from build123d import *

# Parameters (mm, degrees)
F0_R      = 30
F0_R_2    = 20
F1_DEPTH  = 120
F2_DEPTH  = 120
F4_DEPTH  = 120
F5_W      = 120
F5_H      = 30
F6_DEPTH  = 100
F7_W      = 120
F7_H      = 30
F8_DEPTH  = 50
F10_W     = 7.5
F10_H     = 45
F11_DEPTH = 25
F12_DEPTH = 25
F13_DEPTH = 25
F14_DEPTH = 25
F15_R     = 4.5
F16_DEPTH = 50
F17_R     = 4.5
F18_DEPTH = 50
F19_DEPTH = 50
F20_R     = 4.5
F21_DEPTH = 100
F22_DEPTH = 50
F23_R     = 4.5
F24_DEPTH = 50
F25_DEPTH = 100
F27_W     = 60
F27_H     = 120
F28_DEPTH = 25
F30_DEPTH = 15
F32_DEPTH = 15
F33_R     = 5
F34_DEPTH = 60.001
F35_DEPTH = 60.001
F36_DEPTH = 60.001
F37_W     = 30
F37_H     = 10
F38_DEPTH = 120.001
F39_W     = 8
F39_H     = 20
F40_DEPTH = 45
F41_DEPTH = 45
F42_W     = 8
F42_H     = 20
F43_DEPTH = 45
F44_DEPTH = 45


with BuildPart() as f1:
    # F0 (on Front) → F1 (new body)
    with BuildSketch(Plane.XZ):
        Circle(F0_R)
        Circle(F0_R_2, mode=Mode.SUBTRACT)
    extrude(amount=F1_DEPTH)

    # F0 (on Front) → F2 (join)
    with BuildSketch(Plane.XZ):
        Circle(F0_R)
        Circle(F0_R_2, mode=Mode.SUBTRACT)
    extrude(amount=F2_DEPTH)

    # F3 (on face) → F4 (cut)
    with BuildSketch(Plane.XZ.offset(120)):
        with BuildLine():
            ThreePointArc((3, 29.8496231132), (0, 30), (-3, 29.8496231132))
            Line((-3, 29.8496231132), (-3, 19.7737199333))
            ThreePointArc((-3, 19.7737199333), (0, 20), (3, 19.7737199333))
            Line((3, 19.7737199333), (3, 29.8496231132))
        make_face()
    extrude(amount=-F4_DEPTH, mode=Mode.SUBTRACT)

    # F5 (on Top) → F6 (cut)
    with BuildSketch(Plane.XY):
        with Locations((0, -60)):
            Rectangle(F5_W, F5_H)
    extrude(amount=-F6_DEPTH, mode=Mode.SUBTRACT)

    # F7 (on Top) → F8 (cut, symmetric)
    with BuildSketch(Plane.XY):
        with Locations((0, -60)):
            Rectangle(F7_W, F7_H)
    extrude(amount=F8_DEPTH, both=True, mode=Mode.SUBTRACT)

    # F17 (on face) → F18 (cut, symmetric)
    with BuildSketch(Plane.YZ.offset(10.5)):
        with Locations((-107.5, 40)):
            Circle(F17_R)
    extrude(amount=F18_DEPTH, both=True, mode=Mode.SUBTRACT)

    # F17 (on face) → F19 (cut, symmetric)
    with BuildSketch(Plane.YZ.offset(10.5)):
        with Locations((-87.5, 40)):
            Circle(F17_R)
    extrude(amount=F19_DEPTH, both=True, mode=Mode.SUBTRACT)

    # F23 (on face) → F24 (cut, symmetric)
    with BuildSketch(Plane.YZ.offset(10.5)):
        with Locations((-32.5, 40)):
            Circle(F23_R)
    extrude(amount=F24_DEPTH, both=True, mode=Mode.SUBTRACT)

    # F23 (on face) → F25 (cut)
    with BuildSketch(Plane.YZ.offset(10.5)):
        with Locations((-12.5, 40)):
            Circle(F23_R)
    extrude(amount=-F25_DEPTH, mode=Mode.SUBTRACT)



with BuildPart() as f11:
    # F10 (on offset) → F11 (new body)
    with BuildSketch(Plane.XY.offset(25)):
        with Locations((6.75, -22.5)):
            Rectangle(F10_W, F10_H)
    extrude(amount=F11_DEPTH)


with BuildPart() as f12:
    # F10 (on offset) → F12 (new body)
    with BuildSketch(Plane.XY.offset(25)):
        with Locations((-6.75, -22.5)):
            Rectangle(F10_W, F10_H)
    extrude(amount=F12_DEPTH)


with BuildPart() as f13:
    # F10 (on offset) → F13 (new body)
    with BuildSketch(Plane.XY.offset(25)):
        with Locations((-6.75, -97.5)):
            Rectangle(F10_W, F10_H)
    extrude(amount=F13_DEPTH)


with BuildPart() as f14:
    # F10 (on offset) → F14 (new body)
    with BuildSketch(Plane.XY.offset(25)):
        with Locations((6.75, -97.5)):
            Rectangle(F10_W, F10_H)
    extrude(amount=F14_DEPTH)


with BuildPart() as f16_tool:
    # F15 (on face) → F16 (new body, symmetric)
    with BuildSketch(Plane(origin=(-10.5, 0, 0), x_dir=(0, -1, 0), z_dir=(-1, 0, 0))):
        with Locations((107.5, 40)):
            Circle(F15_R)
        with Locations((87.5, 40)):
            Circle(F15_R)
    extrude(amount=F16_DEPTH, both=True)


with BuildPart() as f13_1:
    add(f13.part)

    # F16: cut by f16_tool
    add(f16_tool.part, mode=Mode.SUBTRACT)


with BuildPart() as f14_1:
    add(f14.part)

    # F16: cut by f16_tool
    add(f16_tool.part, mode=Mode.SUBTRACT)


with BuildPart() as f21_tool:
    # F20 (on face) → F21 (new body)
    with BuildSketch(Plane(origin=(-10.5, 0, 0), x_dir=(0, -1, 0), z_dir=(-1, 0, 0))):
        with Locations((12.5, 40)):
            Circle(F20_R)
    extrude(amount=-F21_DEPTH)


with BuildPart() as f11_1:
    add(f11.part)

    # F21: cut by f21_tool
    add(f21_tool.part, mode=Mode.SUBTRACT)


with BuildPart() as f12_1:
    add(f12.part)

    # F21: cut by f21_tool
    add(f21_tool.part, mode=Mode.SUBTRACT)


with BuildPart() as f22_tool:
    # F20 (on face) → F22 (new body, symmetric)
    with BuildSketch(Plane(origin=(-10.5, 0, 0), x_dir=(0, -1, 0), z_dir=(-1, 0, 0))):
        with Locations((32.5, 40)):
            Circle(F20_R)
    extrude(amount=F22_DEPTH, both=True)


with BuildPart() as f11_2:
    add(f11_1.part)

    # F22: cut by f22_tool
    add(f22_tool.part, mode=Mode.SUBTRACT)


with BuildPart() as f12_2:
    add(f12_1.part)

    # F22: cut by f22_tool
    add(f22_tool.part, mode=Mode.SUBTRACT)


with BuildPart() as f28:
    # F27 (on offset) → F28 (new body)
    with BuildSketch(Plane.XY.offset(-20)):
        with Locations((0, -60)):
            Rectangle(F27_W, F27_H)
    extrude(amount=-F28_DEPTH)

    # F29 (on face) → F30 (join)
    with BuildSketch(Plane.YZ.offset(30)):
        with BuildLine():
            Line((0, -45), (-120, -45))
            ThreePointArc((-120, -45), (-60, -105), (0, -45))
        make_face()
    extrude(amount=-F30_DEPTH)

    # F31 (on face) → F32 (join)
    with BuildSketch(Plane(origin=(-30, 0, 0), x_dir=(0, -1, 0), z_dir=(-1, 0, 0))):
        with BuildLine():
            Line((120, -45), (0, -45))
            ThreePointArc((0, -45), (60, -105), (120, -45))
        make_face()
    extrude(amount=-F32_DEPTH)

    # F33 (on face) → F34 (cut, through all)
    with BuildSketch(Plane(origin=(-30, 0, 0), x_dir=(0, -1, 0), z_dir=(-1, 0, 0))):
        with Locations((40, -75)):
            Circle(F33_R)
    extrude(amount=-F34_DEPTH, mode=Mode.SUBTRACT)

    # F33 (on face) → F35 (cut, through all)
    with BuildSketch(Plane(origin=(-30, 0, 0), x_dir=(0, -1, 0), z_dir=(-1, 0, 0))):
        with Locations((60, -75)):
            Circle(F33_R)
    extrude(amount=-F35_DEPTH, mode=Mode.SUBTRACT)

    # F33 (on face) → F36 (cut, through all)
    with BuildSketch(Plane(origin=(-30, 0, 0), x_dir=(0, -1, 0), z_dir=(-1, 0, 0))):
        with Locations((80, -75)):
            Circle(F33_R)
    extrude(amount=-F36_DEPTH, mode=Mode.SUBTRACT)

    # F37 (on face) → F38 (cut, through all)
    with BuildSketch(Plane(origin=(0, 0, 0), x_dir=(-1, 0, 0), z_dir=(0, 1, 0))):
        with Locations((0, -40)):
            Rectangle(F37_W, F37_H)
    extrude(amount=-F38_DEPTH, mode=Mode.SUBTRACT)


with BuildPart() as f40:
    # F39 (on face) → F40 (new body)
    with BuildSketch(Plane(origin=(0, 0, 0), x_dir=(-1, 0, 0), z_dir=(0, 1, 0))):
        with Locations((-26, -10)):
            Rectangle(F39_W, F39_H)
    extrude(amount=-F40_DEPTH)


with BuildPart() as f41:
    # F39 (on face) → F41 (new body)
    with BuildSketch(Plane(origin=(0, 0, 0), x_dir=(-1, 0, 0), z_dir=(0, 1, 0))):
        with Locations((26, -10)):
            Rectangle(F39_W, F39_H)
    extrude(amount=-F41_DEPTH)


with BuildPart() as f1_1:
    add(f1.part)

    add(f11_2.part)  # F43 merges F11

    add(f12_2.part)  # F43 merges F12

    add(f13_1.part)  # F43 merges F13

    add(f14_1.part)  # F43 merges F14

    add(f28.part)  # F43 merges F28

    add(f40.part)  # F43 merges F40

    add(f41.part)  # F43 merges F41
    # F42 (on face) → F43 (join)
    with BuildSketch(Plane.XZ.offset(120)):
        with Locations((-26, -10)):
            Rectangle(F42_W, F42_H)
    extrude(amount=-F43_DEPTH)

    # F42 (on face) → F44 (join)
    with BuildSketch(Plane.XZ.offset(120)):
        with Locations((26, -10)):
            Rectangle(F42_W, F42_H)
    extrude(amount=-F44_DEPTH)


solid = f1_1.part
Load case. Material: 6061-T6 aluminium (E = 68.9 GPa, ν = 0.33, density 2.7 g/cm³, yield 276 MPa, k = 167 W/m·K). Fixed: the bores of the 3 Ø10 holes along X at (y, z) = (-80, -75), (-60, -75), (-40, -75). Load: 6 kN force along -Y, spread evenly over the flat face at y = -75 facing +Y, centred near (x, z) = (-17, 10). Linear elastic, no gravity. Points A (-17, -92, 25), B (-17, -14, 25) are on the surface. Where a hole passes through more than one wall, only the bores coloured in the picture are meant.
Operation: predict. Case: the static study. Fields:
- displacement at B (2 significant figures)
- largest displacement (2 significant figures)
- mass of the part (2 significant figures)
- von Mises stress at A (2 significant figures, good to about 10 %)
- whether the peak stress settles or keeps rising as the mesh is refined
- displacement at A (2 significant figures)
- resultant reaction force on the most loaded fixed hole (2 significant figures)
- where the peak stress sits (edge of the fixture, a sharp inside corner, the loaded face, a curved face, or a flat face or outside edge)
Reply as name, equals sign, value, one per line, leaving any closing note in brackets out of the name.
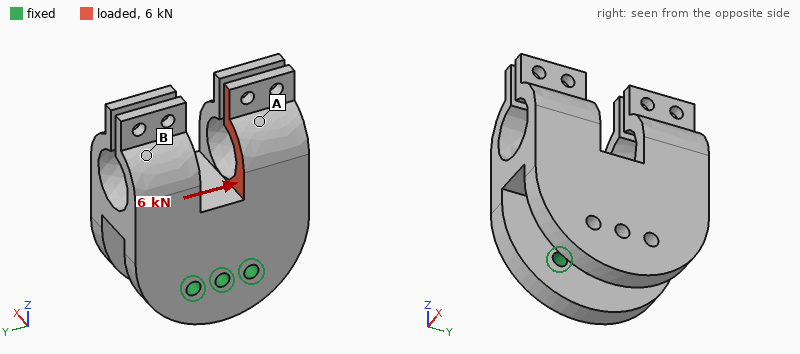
displacement at B = 0.047 mm
largest displacement = 0.22 mm
mass of the part = 1.2 kg
von Mises stress at A = 14 MPa
whether the peak stress settles or keeps rising as the mesh is refined = keeps rising
displacement at A = 0.13 mm
resultant reaction force on the most loaded fixed hole = 11 kN
where the peak stress sits = edge of the fixture
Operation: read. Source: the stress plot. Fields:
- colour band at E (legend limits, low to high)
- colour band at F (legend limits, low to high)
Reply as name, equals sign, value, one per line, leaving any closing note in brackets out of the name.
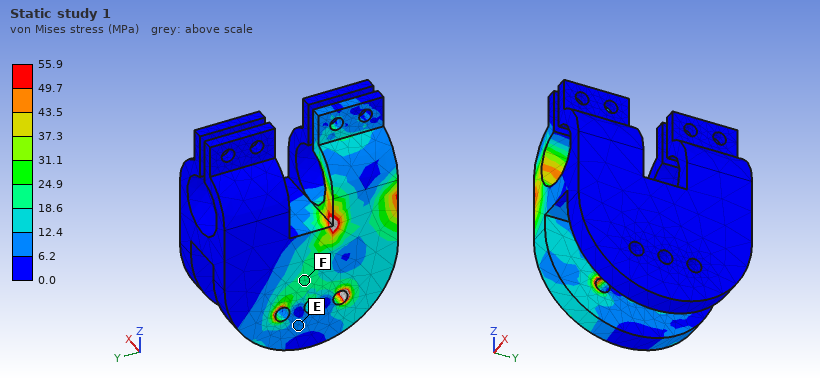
colour band at E = 6.2 to 12.4 MPa
colour band at F = 18.6 to 24.9 MPa
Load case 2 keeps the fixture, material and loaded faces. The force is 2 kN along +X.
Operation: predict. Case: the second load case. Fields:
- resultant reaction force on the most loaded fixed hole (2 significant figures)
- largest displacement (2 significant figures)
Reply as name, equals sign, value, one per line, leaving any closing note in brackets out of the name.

resultant reaction force on the most loaded fixed hole = 990 N
largest displacement = 0.58 mm
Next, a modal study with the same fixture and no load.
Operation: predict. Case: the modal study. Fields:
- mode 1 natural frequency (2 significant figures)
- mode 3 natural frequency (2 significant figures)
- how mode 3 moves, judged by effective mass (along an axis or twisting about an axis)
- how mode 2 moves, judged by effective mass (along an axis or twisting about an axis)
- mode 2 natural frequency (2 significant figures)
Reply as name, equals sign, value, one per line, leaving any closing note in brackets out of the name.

mode 1 natural frequency = 590 Hz
mode 3 natural frequency = 1500 Hz
how mode 3 moves, judged by effective mass = along X
how mode 2 moves, judged by effective mass = along Y
mode 2 natural frequency = 1000 Hz
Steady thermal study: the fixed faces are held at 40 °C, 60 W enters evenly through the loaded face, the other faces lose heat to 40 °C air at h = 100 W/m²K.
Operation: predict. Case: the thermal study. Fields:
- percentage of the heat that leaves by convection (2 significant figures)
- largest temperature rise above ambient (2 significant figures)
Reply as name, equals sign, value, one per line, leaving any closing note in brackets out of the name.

percentage of the heat that leaves by convection = 59 %
largest temperature rise above ambient = 32 K
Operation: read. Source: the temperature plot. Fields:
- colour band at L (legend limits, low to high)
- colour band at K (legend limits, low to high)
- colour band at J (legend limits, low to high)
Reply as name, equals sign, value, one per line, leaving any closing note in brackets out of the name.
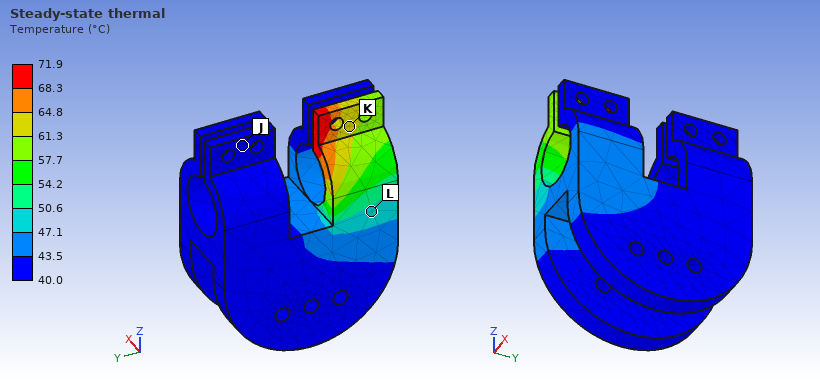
colour band at L = 47.1 to 50.6 °C
colour band at K = 61.3 to 64.8 °C
colour band at J = 40.0 to 43.5 °C
